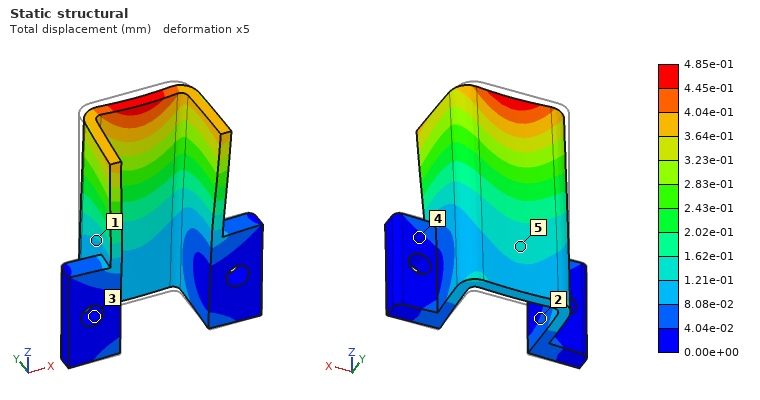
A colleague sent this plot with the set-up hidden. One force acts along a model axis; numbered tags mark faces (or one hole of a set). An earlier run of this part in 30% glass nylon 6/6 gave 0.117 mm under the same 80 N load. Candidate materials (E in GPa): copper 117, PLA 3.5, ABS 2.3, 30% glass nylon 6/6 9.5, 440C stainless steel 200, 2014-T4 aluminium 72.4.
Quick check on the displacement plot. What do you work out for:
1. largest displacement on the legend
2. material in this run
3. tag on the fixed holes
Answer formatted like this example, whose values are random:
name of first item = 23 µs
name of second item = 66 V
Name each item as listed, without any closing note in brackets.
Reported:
largest displacement on the legend = 4.85e-01 mm
material in this run = ABS
tag on the fixed holes = 3
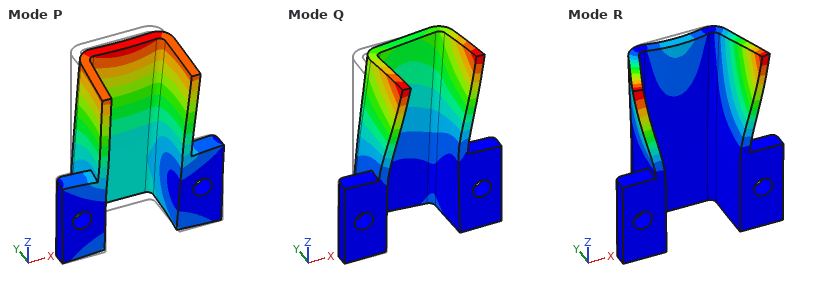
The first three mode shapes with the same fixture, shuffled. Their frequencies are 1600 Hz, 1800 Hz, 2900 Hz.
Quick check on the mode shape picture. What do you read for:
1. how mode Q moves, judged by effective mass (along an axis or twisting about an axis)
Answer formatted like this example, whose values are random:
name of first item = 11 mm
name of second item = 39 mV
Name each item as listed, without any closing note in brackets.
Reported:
how mode Q moves, judged by effective mass = along X
